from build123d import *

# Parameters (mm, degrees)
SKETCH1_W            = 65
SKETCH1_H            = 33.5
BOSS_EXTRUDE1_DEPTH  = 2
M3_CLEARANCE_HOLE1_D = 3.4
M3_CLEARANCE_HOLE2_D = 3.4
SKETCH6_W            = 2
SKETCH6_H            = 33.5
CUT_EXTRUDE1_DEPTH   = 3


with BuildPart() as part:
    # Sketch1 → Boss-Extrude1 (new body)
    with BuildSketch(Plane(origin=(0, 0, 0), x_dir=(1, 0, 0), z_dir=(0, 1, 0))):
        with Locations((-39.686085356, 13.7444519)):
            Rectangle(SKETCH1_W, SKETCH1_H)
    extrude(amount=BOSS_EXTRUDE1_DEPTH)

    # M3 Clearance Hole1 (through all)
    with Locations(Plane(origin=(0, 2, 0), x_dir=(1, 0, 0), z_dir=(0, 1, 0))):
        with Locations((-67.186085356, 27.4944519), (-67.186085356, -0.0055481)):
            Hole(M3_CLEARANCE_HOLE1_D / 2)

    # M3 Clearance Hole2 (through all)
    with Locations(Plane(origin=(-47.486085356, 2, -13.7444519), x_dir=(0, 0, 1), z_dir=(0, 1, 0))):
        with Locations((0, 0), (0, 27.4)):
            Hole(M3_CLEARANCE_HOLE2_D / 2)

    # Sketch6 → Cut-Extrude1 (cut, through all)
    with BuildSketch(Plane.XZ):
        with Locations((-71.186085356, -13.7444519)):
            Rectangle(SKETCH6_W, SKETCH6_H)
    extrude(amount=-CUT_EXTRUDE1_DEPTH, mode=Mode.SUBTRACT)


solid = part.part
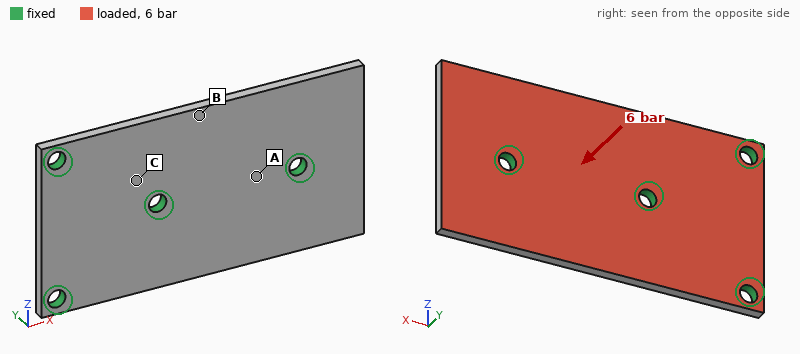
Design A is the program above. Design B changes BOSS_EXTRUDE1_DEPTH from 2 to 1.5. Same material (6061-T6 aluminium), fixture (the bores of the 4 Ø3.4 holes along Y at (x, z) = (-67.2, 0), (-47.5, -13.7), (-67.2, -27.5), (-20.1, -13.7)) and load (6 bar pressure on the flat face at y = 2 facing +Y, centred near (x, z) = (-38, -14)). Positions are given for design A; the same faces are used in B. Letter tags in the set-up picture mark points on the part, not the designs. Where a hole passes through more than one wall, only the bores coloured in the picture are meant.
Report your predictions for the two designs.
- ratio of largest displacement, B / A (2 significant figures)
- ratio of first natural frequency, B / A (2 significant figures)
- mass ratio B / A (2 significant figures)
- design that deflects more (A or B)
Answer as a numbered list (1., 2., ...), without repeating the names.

1. 2.3
2. 0.77
3. 0.75
4. B
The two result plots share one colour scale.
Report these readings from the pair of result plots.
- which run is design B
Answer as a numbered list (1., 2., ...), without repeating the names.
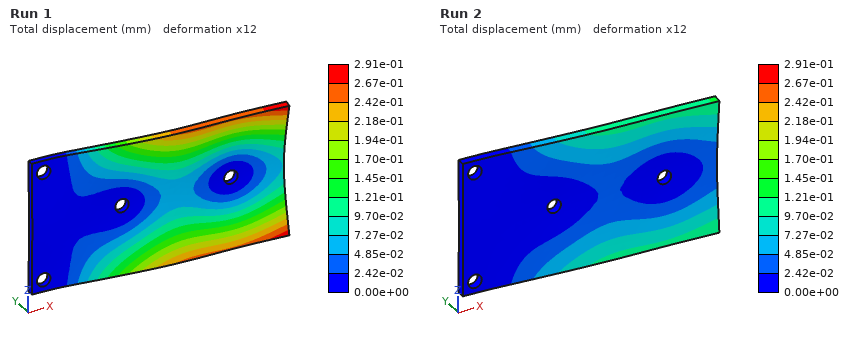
1. Run 1
